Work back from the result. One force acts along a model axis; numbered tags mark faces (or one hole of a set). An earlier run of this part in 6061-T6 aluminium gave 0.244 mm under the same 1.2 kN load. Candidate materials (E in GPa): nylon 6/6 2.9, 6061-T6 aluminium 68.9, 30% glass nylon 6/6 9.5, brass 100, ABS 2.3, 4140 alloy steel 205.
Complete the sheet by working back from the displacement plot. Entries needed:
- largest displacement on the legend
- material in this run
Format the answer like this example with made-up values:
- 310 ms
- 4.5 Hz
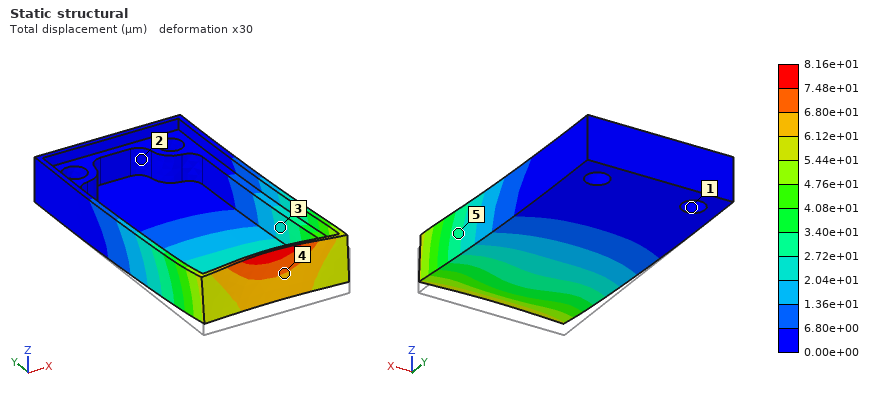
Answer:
- 8.16e+01 µm
- 4140 alloy steel
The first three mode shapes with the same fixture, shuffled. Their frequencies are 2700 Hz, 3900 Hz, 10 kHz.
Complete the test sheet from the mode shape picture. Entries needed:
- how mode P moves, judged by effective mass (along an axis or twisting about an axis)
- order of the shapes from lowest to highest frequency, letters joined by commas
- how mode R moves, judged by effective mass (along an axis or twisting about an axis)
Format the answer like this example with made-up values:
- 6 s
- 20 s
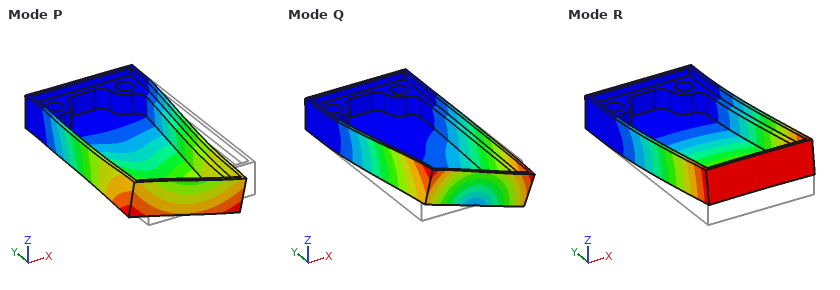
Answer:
- along X
- R, Q, P
- along Z
